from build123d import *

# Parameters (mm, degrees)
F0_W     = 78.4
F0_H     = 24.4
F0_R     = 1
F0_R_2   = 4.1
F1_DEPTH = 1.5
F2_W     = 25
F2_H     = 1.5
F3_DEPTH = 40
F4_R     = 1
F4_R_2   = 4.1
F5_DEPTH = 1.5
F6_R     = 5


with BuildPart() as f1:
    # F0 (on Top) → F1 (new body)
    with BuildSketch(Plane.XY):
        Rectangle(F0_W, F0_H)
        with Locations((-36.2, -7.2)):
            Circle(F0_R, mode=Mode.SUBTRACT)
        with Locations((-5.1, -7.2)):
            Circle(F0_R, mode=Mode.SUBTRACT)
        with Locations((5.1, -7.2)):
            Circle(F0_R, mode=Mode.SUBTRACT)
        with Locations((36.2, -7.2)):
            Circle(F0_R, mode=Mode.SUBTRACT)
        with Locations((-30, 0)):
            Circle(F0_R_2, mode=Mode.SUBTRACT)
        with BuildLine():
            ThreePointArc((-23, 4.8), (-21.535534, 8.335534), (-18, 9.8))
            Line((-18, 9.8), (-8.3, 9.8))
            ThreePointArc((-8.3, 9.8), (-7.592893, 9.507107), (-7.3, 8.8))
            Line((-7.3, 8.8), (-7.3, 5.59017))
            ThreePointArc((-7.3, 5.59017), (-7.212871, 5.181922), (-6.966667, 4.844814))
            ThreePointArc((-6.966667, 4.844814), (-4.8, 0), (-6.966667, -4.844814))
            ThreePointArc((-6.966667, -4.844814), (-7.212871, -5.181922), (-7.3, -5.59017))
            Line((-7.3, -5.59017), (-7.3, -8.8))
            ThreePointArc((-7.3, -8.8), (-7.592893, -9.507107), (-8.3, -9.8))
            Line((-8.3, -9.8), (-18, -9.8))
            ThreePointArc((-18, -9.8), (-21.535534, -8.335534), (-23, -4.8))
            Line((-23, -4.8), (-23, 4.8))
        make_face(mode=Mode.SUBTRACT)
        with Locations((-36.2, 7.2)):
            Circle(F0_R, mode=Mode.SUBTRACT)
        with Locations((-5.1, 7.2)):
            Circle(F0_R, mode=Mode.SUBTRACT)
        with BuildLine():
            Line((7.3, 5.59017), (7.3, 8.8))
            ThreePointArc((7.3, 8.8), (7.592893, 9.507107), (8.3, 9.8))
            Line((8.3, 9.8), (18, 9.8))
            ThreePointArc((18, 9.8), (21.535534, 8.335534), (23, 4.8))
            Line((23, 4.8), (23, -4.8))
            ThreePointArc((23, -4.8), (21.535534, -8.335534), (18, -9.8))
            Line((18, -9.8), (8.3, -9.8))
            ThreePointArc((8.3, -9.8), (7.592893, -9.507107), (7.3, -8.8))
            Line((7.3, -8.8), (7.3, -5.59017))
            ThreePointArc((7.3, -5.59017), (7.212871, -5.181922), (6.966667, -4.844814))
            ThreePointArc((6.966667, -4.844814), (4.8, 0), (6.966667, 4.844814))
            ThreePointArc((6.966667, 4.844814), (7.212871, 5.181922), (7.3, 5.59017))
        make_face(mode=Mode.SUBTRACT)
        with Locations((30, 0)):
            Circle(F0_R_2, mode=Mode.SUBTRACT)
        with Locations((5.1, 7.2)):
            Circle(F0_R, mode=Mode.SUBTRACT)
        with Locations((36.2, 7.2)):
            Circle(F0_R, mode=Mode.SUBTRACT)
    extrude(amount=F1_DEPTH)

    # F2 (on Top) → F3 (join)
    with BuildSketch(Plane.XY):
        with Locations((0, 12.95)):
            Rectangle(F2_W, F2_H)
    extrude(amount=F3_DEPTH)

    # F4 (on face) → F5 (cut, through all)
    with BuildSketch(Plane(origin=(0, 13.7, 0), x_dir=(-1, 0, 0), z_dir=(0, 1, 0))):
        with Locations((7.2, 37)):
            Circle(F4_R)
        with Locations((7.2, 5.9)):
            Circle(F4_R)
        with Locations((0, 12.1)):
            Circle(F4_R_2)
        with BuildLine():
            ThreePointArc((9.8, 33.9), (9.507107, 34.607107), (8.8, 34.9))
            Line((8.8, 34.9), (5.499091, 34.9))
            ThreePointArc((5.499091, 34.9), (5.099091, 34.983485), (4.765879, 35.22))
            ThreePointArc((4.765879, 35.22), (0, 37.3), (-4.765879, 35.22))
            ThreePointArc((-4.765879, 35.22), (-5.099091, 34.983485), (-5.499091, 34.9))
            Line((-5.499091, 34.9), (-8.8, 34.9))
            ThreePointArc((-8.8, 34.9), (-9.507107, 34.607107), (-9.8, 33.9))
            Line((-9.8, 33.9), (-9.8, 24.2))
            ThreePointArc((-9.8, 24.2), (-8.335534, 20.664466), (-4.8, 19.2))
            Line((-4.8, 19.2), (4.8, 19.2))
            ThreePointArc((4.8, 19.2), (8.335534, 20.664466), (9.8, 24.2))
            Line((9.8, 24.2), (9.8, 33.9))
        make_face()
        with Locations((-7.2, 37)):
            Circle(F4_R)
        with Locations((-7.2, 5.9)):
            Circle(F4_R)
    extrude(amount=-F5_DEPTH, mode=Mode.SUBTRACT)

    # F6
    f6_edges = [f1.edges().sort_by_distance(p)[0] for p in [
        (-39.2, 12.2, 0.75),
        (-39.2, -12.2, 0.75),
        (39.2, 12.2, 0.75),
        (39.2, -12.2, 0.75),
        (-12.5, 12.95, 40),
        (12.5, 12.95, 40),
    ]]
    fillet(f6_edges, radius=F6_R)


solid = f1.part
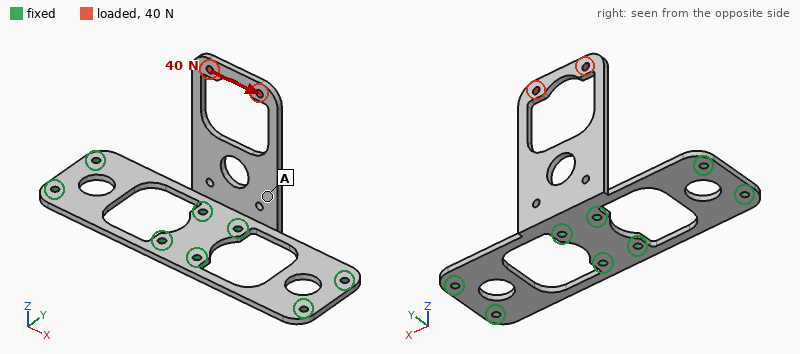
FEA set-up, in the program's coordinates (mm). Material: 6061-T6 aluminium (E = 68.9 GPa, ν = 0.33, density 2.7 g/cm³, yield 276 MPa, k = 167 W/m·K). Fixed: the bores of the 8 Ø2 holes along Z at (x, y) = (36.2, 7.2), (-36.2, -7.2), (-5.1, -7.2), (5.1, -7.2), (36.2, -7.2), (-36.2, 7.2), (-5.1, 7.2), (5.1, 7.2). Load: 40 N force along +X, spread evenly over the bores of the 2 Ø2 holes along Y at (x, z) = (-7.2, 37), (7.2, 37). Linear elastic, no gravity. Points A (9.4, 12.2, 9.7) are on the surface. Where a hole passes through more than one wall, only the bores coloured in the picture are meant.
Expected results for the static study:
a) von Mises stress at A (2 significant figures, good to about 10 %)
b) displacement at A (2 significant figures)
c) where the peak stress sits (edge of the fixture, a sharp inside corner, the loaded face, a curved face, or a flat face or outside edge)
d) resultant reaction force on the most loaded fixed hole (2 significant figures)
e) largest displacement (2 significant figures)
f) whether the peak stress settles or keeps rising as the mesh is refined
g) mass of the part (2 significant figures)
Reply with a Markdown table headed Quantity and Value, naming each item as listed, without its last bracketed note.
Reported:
| Quantity | Value |
|---|---|
| von Mises stress at A | 18 MPa |
| displacement at A | 0.054 mm |
| where the peak stress sits | edge of the fixture |
| resultant reaction force on the most loaded fixed hole | 110 N |
| largest displacement | 0.21 mm |
| whether the peak stress settles or keeps rising as the mesh is refined | keeps rising |
| mass of the part | 7.1 g |
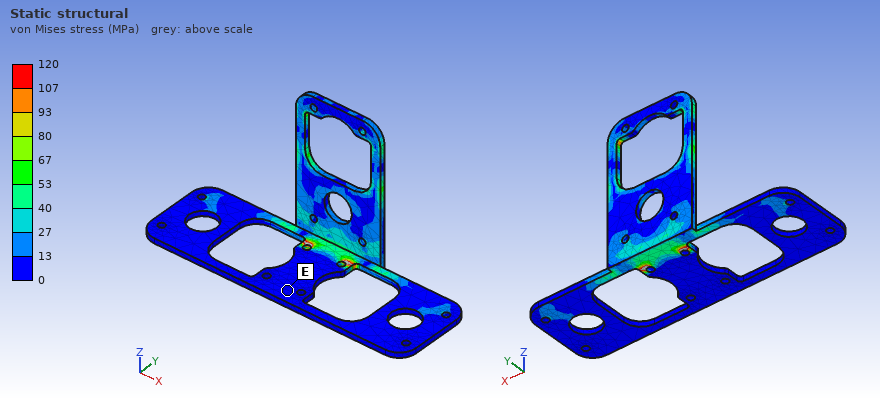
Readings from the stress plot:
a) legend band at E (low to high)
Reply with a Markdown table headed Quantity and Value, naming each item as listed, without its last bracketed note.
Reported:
| Quantity | Value |
|---|---|
| legend band at E | 0 to 13 MPa |
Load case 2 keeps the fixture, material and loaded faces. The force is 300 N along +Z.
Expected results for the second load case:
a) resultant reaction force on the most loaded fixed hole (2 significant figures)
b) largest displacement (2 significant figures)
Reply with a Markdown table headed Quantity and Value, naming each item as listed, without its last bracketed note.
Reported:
| Quantity | Value |
|---|---|
| resultant reaction force on the most loaded fixed hole | 150 N |
| largest displacement | 0.53 mm |
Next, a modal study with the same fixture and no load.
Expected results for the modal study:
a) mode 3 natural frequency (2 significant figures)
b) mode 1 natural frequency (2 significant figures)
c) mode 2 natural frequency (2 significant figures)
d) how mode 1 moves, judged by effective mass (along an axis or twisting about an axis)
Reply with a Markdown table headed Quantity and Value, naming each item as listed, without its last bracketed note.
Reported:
| Quantity | Value |
|---|---|
| mode 3 natural frequency | 2900 Hz |
| mode 1 natural frequency | 780 Hz |
| mode 2 natural frequency | 2200 Hz |
| how mode 1 moves, judged by effective mass | along Y |
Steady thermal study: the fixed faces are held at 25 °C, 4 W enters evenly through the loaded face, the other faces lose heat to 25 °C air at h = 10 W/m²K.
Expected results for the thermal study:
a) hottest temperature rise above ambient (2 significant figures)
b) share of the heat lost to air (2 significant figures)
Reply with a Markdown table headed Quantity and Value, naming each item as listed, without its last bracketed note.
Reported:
| Quantity | Value |
|---|---|
| hottest temperature rise above ambient | 72 K |
| share of the heat lost to air | 10 % |
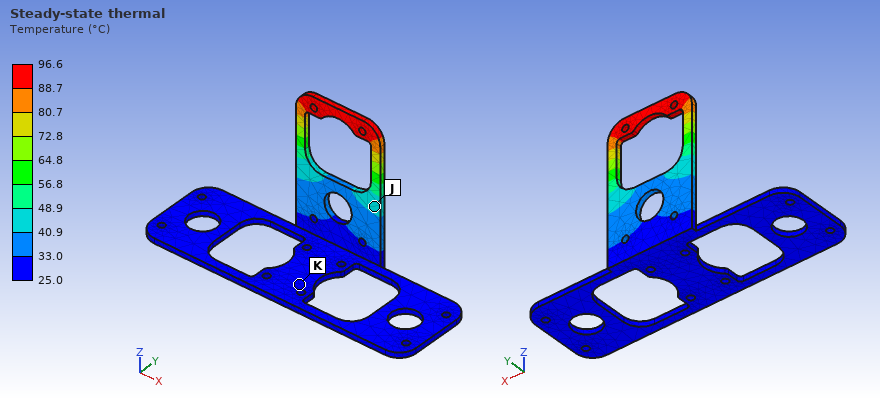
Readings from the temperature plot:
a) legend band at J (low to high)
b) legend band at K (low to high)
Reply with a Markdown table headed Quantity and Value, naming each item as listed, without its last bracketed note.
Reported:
| Quantity | Value |
|---|---|
| legend band at J | 40.9 to 48.9 °C |
| legend band at K | 25.0 to 33.0 °C |
